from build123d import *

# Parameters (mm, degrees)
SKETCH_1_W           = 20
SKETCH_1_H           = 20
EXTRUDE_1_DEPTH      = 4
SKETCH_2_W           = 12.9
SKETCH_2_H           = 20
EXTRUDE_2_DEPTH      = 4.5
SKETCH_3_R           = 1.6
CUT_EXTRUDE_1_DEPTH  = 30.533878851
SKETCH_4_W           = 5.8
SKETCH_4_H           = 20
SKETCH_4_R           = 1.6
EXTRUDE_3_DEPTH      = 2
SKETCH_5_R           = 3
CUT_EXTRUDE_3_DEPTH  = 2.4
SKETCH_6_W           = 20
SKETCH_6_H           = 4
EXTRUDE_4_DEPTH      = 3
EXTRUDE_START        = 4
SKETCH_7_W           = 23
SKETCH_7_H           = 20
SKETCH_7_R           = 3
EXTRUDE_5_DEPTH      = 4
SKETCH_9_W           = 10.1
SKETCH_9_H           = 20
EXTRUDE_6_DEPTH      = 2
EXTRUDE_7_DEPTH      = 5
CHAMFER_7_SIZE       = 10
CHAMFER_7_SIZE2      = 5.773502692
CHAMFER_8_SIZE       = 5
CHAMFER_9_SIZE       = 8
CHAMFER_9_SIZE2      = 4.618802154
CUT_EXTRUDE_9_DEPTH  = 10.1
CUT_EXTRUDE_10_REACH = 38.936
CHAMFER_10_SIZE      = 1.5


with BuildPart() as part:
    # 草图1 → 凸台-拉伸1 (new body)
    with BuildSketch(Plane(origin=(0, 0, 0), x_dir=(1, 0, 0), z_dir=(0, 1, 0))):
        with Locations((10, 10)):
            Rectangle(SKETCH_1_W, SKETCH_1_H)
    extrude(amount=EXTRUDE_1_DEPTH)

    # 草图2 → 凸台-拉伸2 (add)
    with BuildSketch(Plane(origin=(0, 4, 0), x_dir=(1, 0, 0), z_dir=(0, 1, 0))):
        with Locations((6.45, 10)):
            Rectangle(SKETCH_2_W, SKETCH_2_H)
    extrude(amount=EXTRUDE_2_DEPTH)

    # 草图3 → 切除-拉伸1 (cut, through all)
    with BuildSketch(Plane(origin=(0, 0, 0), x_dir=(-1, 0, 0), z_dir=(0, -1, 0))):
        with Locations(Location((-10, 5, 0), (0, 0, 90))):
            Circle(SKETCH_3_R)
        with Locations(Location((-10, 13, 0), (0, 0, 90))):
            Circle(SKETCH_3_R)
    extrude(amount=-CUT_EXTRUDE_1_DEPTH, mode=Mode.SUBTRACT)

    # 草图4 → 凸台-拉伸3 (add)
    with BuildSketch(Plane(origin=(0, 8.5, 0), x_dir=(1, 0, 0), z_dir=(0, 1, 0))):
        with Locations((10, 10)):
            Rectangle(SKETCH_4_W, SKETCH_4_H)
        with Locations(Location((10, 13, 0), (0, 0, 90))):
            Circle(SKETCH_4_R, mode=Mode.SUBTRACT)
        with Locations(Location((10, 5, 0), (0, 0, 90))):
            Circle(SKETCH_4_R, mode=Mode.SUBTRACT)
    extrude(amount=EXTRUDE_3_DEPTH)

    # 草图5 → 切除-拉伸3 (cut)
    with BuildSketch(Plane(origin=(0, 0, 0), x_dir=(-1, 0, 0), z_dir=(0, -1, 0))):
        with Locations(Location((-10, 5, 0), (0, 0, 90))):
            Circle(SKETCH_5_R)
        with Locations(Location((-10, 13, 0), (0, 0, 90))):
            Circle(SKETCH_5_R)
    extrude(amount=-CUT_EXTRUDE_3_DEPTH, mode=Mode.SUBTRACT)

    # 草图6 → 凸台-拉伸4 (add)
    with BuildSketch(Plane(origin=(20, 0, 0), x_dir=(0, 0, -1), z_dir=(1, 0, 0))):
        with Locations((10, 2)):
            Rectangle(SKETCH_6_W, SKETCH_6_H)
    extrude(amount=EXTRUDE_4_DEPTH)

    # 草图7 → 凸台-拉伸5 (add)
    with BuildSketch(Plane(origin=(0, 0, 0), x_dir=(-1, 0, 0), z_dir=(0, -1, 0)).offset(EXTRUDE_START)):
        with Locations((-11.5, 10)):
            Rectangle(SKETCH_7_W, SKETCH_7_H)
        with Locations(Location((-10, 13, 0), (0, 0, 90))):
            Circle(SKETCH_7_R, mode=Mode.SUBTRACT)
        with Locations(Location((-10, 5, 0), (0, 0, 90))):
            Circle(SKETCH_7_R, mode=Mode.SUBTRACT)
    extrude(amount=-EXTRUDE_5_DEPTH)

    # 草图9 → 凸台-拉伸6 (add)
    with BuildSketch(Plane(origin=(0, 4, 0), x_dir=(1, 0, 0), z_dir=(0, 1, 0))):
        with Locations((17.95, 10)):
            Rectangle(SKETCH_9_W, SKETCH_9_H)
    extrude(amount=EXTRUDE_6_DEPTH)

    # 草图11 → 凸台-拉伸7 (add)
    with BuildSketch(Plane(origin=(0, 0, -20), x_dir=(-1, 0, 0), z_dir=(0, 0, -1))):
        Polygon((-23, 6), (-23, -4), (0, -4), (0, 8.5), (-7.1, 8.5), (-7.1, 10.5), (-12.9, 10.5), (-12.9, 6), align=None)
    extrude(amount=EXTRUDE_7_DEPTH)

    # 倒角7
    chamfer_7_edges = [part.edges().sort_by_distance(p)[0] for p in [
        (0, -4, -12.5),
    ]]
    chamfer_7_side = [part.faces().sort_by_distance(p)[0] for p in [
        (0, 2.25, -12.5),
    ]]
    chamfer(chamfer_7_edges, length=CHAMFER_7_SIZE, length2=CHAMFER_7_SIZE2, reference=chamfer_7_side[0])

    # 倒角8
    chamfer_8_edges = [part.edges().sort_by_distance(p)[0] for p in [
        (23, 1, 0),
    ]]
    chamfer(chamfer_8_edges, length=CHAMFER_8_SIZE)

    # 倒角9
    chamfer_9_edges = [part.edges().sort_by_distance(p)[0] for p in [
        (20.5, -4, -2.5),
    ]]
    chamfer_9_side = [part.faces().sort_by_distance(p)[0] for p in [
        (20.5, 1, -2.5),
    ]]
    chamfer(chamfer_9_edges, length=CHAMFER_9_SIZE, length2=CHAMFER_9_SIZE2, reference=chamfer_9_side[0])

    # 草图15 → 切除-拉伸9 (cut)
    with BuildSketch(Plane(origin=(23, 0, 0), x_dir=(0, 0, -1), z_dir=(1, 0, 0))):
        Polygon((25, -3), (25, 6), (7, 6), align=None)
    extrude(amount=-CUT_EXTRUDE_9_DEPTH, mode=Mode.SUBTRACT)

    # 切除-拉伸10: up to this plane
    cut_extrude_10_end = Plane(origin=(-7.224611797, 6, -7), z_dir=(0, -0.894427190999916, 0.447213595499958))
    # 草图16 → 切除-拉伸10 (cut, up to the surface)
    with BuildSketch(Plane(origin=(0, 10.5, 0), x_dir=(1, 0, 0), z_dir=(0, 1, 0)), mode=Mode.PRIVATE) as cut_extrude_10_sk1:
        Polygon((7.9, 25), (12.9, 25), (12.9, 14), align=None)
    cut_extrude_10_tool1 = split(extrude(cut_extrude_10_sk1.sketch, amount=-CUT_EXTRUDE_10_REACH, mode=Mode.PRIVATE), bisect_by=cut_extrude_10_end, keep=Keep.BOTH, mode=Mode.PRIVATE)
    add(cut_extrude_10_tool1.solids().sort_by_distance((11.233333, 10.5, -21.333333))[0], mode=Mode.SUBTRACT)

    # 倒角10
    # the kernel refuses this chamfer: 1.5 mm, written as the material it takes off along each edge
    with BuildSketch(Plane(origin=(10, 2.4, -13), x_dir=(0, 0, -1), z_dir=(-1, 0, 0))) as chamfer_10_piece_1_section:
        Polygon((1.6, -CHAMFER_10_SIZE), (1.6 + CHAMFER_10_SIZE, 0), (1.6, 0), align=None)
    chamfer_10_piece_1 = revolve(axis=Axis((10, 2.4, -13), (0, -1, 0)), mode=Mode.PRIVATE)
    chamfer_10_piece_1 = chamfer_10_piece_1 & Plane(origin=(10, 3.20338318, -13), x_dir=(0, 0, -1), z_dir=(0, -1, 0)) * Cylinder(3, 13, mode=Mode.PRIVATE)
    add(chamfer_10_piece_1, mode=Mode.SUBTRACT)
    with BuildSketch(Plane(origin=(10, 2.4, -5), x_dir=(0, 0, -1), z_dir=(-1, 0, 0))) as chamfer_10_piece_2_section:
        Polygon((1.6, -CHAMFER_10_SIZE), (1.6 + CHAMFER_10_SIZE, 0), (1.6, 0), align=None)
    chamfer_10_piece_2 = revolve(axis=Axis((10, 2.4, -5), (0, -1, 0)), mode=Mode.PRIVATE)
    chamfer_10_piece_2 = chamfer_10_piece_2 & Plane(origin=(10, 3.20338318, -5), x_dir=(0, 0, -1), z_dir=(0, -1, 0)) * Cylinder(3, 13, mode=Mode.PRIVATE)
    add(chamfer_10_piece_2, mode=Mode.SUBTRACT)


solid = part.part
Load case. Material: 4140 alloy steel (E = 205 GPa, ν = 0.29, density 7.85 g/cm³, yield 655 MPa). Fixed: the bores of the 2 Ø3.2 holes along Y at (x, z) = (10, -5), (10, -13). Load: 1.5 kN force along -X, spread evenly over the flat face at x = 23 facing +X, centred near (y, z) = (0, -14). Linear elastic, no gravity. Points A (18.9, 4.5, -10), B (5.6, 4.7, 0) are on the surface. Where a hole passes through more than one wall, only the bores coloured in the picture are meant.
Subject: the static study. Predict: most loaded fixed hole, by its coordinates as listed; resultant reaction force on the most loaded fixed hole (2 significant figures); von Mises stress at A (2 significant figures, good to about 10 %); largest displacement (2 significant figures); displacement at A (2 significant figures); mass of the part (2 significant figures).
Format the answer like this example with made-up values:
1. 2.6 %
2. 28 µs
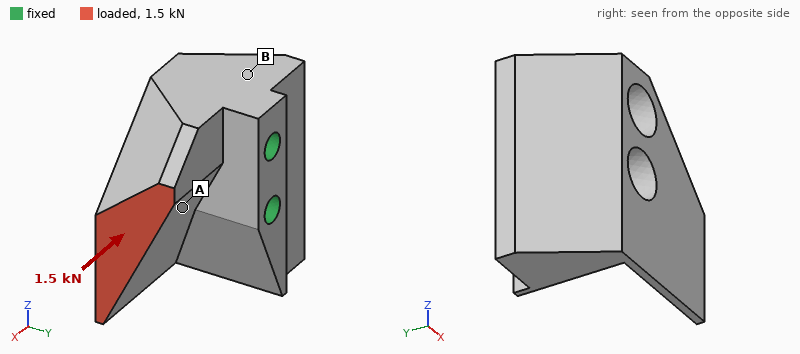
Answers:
1. (10, -13)
2. 1.3 kN
3. 23 MPa
4. 11 µm
5. 4.4 µm
6. 33 g
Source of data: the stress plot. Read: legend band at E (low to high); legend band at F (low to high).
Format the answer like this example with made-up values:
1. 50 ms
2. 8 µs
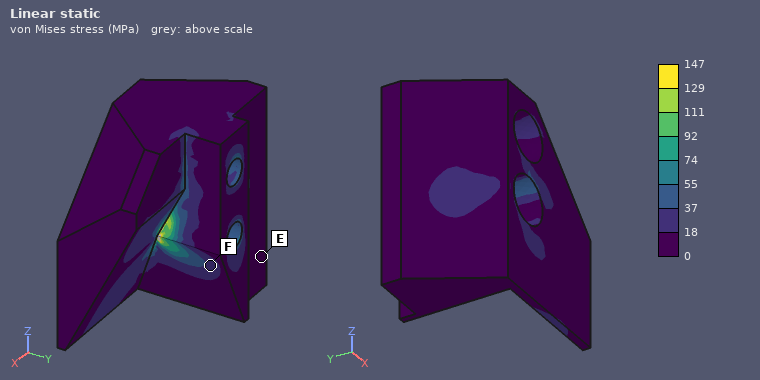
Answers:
1. 0 to 18 MPa
2. 18 to 37 MPa
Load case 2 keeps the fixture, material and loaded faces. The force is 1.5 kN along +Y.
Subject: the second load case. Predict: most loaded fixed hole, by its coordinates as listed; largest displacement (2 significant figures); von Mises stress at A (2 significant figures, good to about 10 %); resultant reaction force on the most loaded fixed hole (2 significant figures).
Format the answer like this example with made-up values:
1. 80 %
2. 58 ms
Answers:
1. (10, -13)
2. 47 µm
3. 75 MPa
4. 1.3 kN
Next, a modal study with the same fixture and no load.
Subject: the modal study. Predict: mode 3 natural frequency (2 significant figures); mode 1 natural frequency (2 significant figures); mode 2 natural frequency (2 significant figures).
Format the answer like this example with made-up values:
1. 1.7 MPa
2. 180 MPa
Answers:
1. 27 kHz
2. 15 kHz
3. 21 kHz
